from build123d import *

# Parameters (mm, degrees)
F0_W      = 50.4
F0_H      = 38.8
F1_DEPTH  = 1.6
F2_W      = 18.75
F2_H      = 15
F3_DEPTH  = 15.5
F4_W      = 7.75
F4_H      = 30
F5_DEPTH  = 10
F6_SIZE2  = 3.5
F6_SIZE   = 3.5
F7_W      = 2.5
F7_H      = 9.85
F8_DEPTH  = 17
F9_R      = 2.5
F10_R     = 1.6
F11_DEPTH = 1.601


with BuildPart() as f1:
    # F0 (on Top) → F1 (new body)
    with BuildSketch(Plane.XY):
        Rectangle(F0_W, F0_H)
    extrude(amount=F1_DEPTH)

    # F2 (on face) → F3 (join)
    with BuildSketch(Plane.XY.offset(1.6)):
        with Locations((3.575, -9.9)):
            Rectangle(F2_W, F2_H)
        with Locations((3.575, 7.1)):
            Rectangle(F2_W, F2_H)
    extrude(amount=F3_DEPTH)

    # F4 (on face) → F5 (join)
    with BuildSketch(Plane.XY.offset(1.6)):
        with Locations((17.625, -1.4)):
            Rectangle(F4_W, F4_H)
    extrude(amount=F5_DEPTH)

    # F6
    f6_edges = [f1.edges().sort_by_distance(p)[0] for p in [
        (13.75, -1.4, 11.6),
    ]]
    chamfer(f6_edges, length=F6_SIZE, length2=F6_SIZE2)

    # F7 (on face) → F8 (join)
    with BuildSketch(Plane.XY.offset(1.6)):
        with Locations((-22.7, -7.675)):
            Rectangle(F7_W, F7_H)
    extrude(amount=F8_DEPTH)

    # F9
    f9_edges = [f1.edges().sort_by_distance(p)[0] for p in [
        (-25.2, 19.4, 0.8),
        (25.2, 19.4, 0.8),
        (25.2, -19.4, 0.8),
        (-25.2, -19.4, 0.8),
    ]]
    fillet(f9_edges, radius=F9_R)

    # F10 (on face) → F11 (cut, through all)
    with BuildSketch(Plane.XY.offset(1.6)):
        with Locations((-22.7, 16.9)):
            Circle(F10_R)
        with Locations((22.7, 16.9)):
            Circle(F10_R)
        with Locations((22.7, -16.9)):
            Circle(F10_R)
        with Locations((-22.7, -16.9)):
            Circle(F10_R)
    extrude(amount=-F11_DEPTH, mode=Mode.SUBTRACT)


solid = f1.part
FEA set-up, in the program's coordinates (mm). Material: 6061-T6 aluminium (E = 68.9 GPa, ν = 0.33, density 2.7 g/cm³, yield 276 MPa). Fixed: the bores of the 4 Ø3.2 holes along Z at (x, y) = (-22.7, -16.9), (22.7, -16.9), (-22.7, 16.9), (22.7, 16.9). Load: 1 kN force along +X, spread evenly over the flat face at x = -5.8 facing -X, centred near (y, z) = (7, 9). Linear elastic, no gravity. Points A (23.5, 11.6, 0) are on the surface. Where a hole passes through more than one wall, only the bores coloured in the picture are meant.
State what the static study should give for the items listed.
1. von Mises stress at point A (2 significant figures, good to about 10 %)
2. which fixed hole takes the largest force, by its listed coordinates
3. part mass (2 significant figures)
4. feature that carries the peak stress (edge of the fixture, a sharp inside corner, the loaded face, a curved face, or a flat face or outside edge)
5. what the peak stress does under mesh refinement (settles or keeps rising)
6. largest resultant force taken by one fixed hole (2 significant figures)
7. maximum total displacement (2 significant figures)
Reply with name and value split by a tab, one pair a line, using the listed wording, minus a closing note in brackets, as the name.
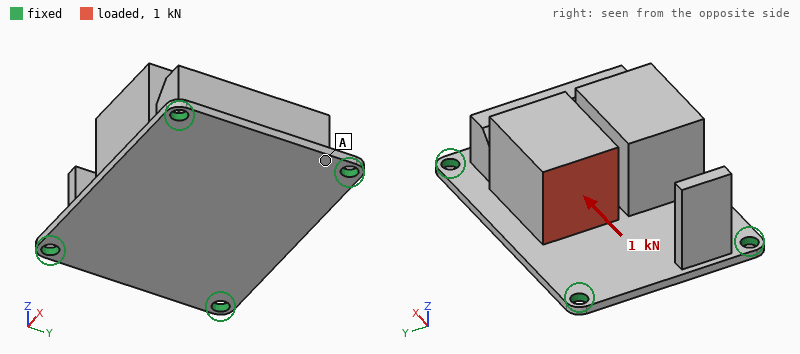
von Mises stress at point A	19 MPa
which fixed hole takes the largest force, by its listed coordinates	(22.7, 16.9)
part mass	39 g
feature that carries the peak stress	edge of the fixture
what the peak stress does under mesh refinement	keeps rising
largest resultant force taken by one fixed hole	380 N
maximum total displacement	0.15 mm
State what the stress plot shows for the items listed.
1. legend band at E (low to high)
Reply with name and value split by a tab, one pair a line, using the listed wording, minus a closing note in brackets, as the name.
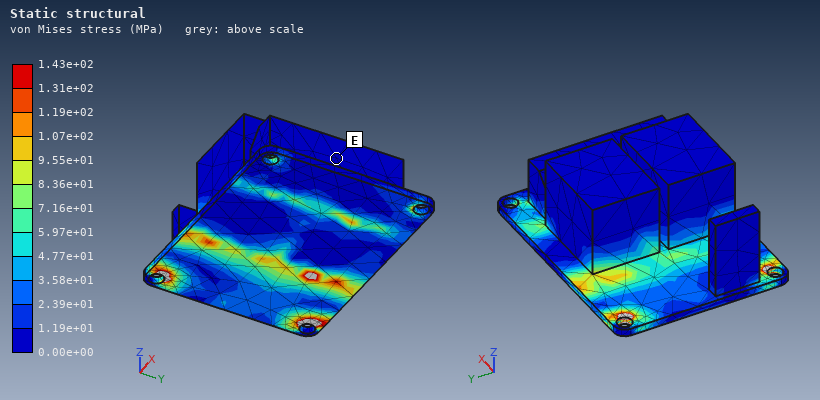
legend band at E	0.00e+00 to 1.19e+01 MPa
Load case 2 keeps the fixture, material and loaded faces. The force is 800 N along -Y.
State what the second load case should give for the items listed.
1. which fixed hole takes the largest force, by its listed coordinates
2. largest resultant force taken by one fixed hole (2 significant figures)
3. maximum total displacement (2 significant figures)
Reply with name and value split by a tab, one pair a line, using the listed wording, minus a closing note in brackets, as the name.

which fixed hole takes the largest force, by its listed coordinates	(22.7, -16.9)
largest resultant force taken by one fixed hole	460 N
maximum total displacement	67 µm
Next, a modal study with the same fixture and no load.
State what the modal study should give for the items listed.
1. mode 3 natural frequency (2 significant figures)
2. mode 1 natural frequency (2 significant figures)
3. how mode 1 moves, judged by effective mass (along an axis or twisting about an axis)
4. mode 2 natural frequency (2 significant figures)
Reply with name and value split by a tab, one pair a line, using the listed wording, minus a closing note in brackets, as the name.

mode 3 natural frequency	4500 Hz
mode 1 natural frequency	2000 Hz
how mode 1 moves, judged by effective mass	along Z
mode 2 natural frequency	4000 Hz
